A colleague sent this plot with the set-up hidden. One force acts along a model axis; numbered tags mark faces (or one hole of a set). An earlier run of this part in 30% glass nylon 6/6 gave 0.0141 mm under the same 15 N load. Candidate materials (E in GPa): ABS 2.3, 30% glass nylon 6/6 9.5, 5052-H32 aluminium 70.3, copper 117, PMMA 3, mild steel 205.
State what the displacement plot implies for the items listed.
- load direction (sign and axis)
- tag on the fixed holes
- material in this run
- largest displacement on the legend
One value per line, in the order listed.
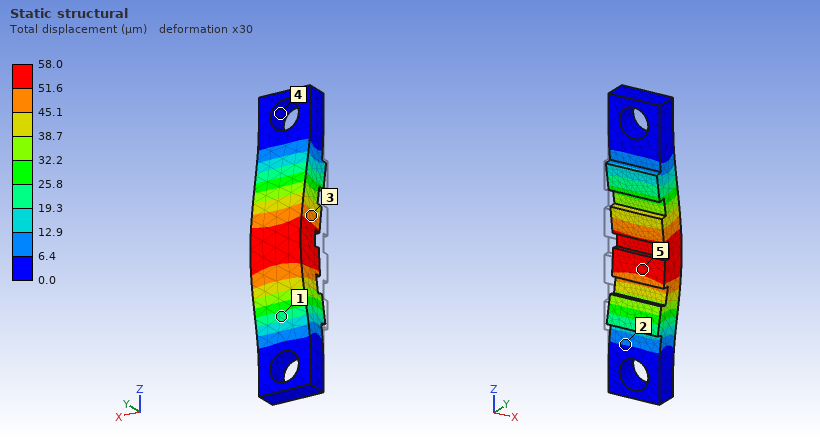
+Y
4
ABS
58.0 µm
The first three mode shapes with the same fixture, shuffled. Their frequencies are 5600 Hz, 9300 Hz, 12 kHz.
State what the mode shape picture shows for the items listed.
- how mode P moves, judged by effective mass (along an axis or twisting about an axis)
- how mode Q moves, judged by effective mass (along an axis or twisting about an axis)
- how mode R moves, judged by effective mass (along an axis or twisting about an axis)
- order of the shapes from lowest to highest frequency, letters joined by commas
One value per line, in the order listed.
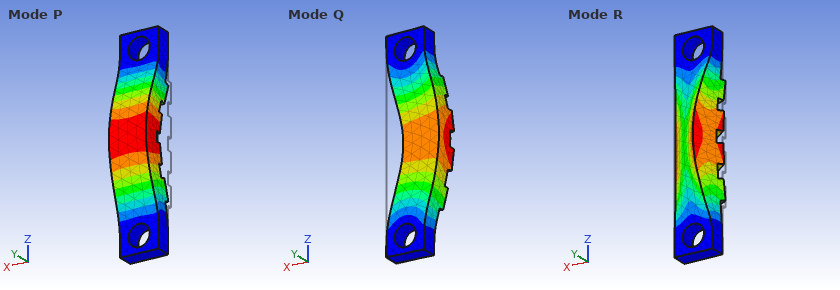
along Y
along X
twisting about Z
P, Q, R
